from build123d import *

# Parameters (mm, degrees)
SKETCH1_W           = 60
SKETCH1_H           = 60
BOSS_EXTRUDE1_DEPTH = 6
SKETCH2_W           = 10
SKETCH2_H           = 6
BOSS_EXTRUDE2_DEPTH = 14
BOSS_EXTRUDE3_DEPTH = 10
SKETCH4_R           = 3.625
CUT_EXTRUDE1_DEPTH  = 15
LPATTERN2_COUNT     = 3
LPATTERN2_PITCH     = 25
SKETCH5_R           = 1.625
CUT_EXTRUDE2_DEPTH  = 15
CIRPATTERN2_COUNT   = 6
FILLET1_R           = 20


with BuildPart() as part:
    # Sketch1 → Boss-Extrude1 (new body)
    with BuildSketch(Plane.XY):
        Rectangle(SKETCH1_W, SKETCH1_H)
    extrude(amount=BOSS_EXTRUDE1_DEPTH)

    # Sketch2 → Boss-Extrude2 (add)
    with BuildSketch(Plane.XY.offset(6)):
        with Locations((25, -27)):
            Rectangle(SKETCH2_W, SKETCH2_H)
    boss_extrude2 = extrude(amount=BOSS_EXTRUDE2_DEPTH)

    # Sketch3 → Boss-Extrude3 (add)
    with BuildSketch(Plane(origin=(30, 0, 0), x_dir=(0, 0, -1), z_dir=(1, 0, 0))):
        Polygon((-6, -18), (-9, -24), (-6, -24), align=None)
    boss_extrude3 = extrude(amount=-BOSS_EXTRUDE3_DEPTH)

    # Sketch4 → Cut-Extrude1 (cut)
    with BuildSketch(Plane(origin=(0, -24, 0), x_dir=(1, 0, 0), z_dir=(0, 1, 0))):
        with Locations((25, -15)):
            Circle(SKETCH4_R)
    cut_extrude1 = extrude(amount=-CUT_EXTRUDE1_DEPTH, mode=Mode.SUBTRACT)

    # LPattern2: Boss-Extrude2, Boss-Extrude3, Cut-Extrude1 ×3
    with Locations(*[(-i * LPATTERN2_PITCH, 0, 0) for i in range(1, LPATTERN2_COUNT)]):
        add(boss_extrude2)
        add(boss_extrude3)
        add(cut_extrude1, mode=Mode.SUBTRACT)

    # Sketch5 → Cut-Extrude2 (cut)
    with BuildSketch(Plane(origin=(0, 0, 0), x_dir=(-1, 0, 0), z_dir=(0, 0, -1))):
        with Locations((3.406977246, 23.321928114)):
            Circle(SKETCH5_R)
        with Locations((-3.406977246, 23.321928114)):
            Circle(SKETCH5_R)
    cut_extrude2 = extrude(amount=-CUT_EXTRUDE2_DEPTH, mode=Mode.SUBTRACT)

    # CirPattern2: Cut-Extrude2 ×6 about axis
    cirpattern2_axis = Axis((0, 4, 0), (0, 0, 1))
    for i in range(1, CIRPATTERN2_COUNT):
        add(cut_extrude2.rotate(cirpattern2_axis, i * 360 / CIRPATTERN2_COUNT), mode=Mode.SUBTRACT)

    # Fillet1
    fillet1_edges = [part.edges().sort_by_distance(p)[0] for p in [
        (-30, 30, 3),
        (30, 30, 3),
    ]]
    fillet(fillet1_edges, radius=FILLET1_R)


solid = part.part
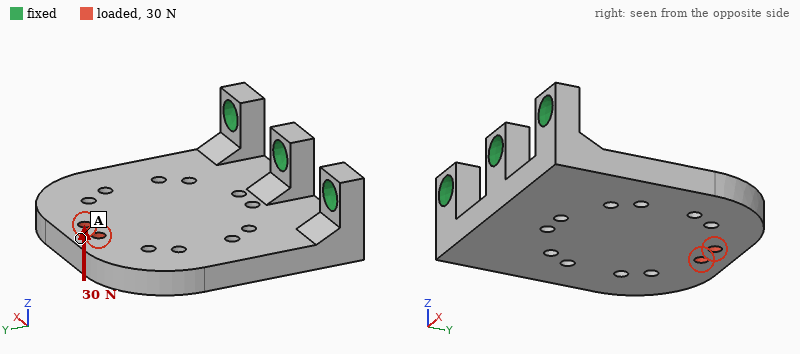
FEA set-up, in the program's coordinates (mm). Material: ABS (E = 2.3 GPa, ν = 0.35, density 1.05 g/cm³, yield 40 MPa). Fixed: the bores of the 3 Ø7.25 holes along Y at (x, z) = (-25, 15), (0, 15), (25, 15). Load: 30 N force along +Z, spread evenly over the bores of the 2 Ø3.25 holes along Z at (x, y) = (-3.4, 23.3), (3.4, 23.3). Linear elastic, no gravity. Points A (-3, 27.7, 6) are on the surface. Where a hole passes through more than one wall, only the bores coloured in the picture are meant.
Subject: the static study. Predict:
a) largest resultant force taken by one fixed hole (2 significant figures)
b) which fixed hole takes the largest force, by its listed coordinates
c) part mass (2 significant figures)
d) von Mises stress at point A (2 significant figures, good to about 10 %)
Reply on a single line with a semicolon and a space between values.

25 N; (0, 15); 23 g; 1.7 MPa
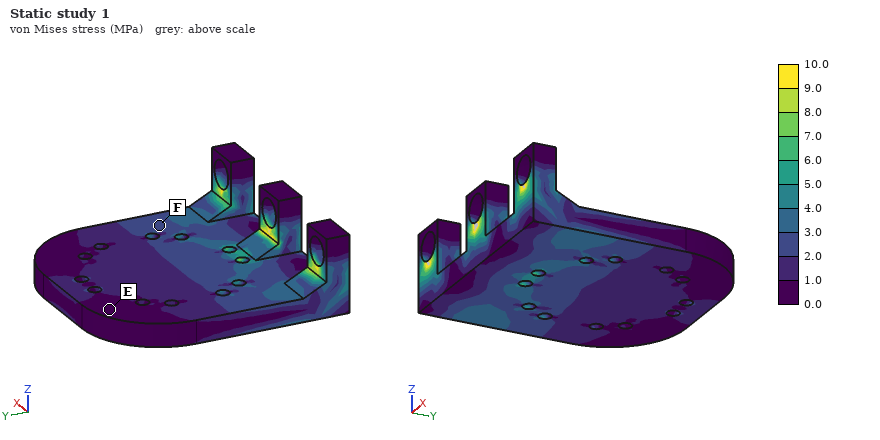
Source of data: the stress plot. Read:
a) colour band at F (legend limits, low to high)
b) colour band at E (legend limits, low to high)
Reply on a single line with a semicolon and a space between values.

2.0 to 3.0 MPa; 0.0 to 1.0 MPa
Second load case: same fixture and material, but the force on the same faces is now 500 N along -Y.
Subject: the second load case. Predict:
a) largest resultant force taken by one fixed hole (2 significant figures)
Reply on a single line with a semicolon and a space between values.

170 N
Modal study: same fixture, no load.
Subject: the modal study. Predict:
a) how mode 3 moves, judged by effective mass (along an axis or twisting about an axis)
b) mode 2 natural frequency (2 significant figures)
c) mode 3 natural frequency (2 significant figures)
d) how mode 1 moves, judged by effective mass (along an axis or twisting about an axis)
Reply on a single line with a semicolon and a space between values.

along X; 1000 Hz; 1700 Hz; along Z
